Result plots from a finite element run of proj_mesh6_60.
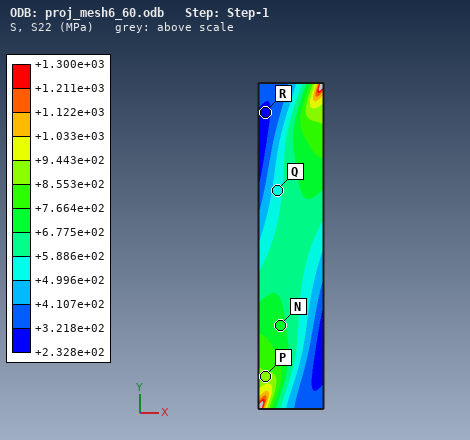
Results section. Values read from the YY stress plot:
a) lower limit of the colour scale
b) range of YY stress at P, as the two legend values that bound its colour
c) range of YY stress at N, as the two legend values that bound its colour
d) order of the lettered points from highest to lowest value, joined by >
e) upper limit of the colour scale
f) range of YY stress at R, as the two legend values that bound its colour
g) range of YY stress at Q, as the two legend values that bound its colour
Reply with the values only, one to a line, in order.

+2.328e+02 MPa
+8.553e+02 to +9.443e+02 MPa
+6.775e+02 to +7.664e+02 MPa
P > N > Q > R
+1.300e+03 MPa
+2.328e+02 to +3.218e+02 MPa
+4.996e+02 to +5.886e+02 MPa
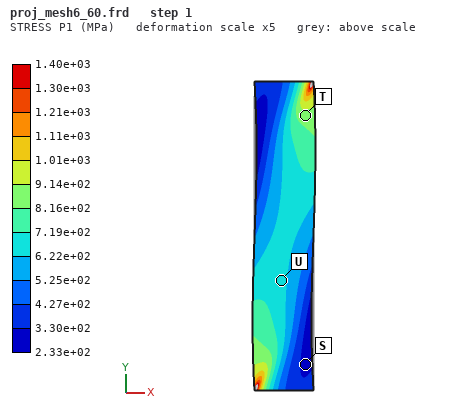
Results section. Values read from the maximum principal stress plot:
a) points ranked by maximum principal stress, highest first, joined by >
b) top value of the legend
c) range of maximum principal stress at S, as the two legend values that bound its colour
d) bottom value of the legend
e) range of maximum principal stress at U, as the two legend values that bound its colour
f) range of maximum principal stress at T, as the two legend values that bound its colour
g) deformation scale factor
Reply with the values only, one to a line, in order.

T > U > S
1.40e+03 MPa
2.33e+02 to 3.30e+02 MPa
2.33e+02 MPa
6.22e+02 to 7.19e+02 MPa
8.16e+02 to 9.14e+02 MPa
5
